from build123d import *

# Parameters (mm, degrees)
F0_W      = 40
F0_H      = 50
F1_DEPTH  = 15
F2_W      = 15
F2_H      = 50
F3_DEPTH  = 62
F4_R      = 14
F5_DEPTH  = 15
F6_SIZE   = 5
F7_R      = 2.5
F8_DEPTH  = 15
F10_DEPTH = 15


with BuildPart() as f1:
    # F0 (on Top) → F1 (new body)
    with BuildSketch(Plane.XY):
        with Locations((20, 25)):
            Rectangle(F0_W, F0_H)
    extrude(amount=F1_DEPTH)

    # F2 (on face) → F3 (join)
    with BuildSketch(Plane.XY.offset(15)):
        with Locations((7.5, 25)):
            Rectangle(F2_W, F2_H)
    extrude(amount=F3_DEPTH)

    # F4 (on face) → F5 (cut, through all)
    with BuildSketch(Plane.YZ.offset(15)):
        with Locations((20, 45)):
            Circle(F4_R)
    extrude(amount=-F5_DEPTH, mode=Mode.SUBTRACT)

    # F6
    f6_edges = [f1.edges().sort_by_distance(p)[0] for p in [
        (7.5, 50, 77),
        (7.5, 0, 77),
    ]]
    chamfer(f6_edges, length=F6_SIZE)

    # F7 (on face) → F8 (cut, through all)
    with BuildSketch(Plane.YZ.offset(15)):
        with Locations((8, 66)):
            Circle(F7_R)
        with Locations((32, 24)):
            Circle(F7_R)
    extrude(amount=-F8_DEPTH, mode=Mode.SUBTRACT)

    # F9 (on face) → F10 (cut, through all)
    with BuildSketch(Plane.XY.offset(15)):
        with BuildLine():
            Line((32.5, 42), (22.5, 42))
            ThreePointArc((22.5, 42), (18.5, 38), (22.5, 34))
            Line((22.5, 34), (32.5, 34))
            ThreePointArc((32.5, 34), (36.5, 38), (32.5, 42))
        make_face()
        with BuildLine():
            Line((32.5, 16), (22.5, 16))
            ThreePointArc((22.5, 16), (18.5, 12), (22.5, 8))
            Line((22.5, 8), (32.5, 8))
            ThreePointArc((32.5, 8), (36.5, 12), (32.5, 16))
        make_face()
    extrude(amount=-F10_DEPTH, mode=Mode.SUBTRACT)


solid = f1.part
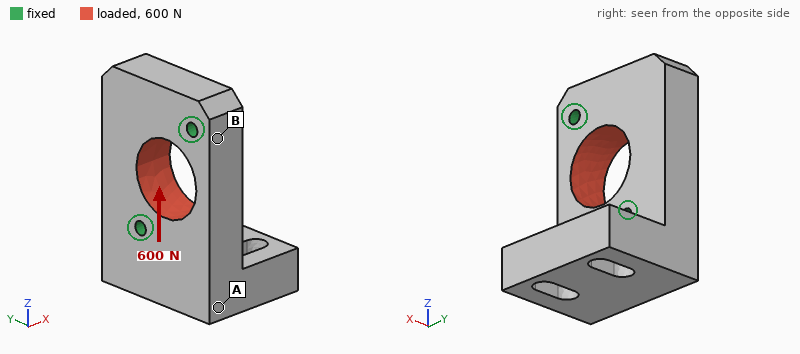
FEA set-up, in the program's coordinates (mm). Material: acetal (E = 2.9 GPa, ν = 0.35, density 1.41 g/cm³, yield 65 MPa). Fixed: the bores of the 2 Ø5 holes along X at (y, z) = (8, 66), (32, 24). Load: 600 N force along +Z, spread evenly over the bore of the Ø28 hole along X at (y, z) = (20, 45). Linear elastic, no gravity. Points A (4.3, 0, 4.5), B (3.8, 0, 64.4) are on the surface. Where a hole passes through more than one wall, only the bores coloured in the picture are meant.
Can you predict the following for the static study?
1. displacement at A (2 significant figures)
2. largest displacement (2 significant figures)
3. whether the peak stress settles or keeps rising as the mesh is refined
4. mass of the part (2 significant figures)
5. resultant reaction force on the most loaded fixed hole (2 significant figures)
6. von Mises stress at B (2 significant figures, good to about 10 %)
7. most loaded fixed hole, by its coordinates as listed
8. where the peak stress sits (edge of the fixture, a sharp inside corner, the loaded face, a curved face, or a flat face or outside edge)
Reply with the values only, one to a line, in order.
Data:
13 µm
13 µm
keeps rising
88 g
320 N
0.62 MPa
(32, 24)
edge of the fixture
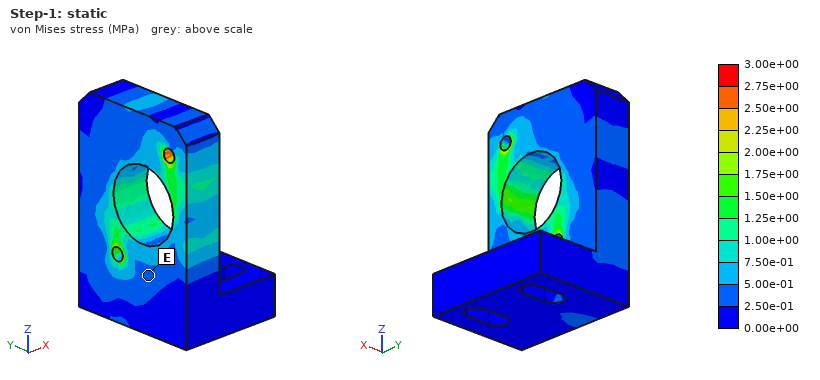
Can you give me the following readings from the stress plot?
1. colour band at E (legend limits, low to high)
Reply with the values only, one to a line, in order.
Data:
2.50e-01 to 5.00e-01 MPa
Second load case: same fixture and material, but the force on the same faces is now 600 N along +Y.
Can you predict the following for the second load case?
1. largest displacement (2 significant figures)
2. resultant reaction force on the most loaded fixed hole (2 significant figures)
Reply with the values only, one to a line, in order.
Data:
20 µm
310 N
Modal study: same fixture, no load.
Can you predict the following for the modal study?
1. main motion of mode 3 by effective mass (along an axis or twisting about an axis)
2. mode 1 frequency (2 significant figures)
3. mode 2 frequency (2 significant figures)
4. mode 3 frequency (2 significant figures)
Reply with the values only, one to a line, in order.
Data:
along X
1300 Hz
1700 Hz
2200 Hz
